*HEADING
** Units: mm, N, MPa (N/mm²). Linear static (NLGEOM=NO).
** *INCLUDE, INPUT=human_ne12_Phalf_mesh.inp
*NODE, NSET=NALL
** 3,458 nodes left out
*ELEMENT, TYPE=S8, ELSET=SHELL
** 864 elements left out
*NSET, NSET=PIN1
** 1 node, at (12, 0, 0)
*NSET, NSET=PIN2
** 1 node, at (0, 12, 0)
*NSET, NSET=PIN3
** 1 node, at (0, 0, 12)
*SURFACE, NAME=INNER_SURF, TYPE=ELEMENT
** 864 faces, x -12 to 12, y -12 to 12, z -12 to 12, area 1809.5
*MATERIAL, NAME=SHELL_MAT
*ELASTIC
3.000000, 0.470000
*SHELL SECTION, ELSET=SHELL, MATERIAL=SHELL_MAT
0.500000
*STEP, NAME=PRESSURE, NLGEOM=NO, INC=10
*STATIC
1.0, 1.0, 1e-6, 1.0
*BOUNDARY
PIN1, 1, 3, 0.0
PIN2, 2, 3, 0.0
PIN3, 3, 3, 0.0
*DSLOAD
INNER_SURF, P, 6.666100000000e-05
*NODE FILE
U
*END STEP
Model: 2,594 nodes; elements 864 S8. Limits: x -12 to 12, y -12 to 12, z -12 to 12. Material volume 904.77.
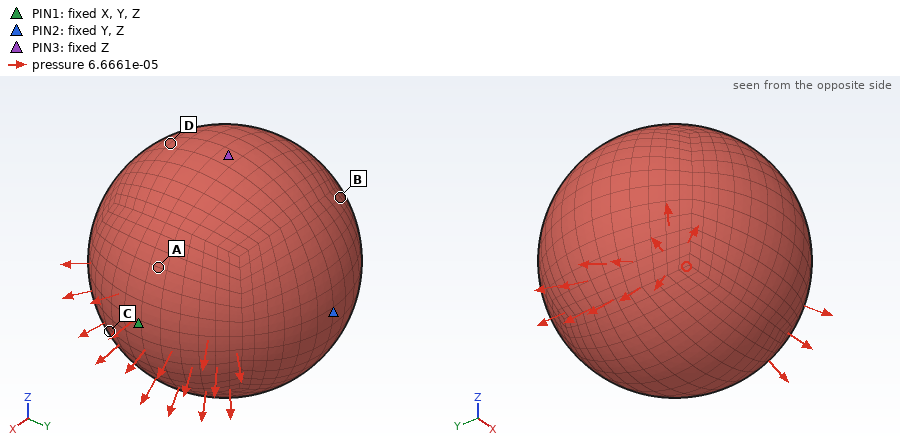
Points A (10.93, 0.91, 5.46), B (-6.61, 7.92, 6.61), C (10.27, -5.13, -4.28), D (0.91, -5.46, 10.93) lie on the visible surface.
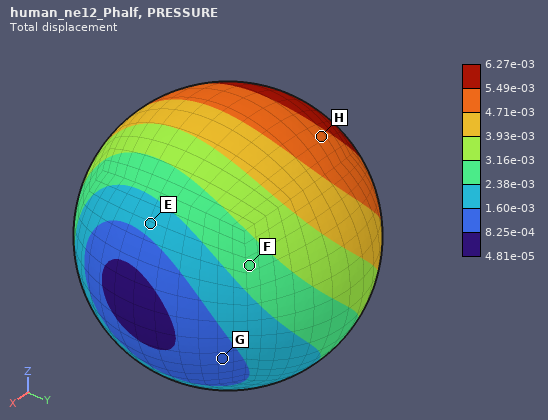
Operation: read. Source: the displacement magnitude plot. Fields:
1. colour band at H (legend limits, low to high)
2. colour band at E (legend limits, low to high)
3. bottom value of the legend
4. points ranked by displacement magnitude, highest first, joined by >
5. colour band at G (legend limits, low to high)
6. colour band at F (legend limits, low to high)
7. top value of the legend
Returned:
4.71e-03 to 5.49e-03
1.60e-03 to 2.38e-03
4.81e-05
H > F > E > G
8.25e-04 to 1.60e-03
2.38e-03 to 3.16e-03
6.27e-03
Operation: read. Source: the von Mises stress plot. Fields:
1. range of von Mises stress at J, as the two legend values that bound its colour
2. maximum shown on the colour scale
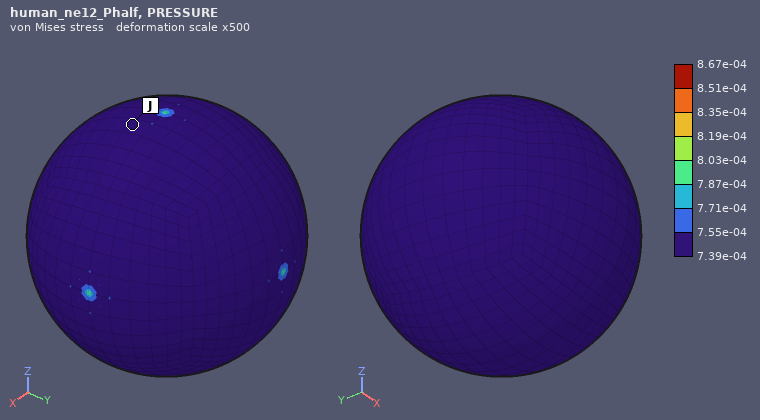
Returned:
7.39e-04 to 7.55e-04
8.67e-04
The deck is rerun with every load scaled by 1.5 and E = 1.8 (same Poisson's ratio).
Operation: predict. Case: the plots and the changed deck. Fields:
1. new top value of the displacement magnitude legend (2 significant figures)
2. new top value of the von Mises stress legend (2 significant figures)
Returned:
0.016
0.0013
